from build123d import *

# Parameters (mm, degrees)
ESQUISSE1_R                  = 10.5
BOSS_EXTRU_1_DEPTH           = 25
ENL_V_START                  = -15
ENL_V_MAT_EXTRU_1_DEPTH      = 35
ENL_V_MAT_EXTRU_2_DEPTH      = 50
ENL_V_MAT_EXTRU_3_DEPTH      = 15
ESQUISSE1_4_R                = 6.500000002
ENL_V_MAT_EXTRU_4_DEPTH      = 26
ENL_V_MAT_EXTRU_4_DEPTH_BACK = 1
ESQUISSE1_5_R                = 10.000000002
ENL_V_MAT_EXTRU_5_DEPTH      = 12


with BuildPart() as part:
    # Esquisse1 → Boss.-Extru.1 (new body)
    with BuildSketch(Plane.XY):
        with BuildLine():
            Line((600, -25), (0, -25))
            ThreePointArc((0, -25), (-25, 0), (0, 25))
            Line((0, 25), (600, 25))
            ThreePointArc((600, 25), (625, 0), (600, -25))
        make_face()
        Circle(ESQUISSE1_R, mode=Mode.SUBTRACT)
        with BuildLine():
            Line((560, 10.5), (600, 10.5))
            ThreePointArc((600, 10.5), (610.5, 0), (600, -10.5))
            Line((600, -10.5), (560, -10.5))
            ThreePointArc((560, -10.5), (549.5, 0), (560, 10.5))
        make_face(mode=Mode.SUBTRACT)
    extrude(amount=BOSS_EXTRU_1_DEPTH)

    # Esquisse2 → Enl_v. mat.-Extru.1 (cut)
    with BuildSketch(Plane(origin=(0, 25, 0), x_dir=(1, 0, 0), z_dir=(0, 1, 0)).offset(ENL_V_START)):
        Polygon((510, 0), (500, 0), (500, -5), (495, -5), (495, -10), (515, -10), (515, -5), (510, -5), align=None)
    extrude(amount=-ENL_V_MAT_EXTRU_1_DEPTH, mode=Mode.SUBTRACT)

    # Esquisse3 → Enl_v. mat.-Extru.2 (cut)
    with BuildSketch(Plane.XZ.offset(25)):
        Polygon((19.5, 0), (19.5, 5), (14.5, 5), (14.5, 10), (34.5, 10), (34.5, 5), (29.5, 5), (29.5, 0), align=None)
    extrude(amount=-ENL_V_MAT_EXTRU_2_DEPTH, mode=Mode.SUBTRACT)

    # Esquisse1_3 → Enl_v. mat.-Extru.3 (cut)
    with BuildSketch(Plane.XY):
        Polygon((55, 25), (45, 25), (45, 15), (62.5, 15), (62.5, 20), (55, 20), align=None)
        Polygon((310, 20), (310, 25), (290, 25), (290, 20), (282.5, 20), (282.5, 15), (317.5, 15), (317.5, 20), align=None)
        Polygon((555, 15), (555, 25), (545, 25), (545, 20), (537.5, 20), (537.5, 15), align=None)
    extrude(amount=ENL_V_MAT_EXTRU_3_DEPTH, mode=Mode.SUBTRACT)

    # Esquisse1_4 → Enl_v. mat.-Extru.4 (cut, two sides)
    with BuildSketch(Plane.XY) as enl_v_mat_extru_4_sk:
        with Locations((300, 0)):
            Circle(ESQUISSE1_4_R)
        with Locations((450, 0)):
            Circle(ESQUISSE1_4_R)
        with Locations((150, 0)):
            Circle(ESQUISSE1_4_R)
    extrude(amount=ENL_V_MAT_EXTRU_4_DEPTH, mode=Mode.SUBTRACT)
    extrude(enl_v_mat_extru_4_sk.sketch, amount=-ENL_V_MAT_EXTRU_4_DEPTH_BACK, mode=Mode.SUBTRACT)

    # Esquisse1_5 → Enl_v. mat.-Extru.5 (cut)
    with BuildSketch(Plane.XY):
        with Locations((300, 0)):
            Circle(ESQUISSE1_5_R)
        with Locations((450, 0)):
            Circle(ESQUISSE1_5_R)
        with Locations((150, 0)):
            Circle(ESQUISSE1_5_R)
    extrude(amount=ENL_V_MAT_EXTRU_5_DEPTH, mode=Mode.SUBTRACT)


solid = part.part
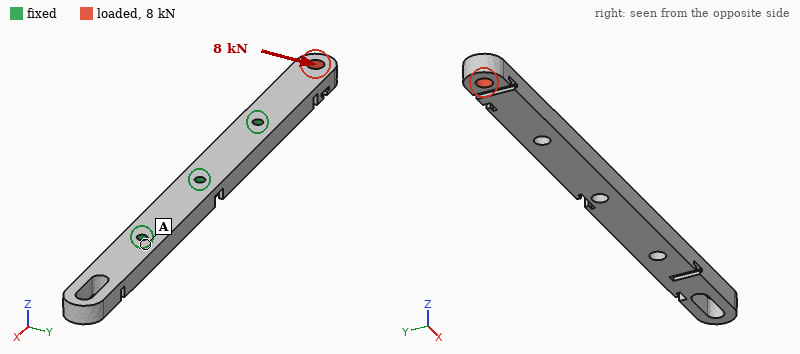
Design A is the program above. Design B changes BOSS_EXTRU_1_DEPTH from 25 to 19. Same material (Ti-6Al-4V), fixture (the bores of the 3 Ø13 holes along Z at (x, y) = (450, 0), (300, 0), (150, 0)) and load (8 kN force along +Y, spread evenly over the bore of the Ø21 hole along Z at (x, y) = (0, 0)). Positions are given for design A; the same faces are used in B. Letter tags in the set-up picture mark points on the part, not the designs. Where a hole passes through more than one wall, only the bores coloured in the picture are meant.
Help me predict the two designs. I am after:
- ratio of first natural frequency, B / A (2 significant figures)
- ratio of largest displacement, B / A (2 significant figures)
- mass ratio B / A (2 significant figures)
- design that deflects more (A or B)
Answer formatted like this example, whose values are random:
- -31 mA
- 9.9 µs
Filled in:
- 0.74
- 1.4
- 0.75
- B
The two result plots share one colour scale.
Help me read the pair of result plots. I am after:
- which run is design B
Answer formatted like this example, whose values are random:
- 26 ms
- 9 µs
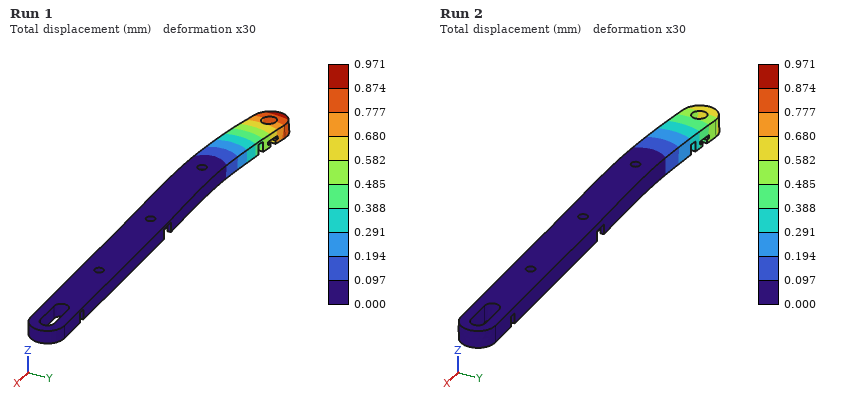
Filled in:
- Run 1
